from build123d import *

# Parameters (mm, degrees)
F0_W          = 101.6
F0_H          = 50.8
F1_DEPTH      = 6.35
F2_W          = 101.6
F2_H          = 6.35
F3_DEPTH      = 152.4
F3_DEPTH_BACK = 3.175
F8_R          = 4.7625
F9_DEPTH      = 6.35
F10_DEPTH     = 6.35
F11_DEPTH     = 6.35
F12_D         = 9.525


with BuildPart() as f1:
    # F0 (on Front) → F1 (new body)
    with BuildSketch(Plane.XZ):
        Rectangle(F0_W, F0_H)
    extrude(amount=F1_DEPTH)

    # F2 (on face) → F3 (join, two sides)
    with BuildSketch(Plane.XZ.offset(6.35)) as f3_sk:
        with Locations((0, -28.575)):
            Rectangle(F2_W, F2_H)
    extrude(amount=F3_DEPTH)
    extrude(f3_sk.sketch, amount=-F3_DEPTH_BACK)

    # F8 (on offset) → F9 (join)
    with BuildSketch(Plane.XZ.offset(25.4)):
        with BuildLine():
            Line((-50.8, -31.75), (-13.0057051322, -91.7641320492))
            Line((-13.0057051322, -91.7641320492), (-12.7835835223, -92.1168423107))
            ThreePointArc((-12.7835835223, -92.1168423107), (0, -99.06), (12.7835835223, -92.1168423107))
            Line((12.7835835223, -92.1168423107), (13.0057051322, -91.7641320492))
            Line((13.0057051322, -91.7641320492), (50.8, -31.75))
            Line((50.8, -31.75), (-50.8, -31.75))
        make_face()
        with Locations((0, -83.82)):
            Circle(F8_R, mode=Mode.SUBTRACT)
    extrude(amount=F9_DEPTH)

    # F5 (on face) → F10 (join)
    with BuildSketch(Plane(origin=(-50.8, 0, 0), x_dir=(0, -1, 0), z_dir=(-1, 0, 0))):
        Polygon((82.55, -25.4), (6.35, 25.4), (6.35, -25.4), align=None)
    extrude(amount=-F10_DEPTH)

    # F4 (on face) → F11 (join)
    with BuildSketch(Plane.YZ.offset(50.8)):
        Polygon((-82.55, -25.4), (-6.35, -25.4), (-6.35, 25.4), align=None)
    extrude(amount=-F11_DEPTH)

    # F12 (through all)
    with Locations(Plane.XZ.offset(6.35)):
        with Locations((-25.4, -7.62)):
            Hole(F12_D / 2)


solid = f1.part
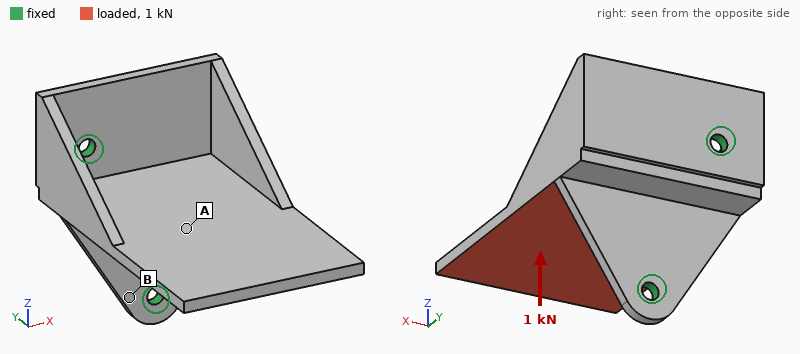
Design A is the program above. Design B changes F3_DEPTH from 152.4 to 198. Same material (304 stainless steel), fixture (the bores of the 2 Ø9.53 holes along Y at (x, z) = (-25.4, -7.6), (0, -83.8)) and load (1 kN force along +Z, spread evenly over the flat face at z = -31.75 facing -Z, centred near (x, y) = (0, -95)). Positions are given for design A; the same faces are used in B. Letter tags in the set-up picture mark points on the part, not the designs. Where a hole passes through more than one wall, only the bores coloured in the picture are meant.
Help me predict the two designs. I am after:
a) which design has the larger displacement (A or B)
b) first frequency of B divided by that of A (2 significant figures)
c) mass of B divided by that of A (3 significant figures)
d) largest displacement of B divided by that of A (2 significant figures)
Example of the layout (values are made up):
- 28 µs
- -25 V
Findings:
- B
- 0.55
- 1.16
- 2.8
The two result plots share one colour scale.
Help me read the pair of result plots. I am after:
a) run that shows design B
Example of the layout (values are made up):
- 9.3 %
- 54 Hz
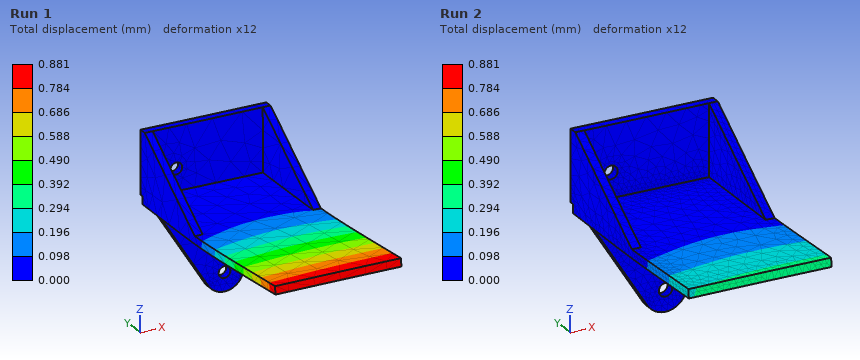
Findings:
- Run 1
